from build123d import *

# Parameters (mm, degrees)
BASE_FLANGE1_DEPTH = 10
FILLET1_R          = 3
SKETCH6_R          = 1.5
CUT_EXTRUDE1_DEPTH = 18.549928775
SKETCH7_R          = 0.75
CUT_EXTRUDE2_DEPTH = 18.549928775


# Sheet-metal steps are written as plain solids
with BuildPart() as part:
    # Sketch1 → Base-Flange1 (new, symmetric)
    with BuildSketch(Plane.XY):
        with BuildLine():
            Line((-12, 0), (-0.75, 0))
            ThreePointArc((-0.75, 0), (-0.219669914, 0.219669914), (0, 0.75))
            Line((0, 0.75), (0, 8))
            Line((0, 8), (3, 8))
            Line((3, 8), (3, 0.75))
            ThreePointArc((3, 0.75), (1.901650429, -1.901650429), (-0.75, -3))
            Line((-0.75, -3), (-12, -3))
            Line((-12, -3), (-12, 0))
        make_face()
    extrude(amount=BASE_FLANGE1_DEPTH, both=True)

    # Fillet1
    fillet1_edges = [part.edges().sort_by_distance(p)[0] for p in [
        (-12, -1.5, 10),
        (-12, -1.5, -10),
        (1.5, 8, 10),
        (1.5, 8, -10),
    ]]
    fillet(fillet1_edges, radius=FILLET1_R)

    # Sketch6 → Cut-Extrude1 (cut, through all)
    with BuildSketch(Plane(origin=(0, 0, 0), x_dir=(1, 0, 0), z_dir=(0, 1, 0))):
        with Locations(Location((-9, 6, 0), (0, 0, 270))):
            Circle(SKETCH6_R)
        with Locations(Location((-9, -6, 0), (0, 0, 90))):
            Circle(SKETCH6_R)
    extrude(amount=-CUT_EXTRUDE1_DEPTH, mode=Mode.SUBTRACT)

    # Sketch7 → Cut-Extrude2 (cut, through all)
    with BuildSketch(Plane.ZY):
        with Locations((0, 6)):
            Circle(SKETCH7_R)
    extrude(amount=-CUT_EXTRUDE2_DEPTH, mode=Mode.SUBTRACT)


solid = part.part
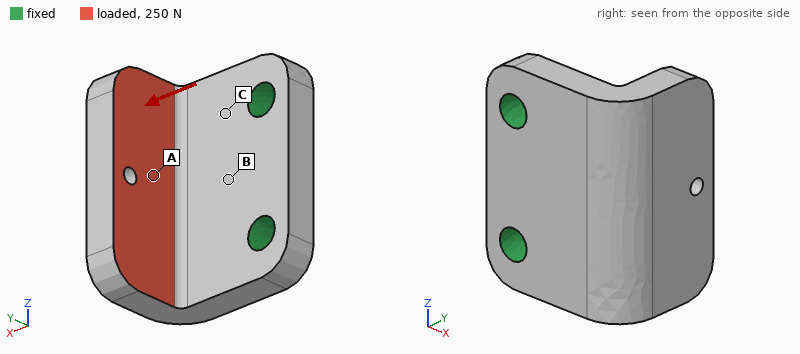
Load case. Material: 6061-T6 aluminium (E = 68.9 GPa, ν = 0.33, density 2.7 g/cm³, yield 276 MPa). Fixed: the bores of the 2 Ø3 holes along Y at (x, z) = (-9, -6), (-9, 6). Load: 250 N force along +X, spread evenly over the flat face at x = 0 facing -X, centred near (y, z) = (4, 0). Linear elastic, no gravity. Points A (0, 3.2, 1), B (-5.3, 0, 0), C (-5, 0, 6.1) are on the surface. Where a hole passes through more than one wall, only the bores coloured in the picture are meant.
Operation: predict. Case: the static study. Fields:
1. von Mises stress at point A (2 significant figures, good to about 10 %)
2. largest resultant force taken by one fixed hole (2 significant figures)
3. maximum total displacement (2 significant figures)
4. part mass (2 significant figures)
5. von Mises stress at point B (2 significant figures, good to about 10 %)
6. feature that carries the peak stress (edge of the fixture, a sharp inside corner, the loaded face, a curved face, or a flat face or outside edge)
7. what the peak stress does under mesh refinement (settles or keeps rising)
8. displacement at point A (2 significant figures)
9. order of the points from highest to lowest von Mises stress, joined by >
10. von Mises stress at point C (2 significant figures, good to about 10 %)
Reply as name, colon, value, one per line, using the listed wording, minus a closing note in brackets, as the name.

von Mises stress at point A: 13 MPa
largest resultant force taken by one fixed hole: 130 N
maximum total displacement: 58 µm
part mass: 3.4 g
von Mises stress at point B: 39 MPa
feature that carries the peak stress: edge of the fixture
what the peak stress does under mesh refinement: keeps rising
displacement at point A: 28 µm
order of the points from highest to lowest von Mises stress, joined by >: C > B > A
von Mises stress at point C: 54 MPa
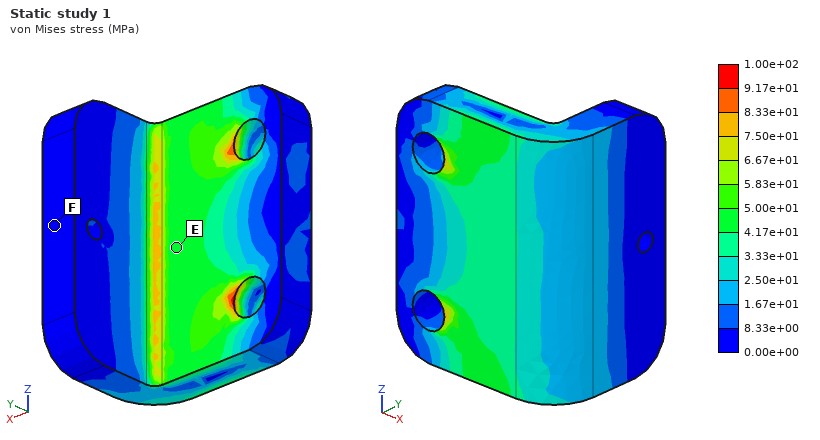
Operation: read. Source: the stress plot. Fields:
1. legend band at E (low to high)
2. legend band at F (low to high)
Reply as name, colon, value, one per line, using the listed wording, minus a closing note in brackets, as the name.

legend band at E: 4.17e+01 to 5.00e+01 MPa
legend band at F: 0.00e+00 to 8.33e+00 MPa
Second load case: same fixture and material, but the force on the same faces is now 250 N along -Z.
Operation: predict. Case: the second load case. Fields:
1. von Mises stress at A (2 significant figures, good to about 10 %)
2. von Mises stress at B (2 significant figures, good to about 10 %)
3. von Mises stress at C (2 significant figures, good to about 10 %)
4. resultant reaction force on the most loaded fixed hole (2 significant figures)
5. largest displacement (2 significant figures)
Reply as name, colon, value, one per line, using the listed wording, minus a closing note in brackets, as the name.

von Mises stress at A: 22 MPa
von Mises stress at B: 26 MPa
von Mises stress at C: 29 MPa
resultant reaction force on the most loaded fixed hole: 220 N
largest displacement: 23 µm
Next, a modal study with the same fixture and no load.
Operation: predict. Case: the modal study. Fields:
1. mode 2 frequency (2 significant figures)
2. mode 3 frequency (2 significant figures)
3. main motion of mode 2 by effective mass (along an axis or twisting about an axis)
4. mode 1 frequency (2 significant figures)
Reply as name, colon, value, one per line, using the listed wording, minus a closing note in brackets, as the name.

mode 2 frequency: 15 kHz
mode 3 frequency: 25 kHz
main motion of mode 2 by effective mass: along Z
mode 1 frequency: 8900 Hz
